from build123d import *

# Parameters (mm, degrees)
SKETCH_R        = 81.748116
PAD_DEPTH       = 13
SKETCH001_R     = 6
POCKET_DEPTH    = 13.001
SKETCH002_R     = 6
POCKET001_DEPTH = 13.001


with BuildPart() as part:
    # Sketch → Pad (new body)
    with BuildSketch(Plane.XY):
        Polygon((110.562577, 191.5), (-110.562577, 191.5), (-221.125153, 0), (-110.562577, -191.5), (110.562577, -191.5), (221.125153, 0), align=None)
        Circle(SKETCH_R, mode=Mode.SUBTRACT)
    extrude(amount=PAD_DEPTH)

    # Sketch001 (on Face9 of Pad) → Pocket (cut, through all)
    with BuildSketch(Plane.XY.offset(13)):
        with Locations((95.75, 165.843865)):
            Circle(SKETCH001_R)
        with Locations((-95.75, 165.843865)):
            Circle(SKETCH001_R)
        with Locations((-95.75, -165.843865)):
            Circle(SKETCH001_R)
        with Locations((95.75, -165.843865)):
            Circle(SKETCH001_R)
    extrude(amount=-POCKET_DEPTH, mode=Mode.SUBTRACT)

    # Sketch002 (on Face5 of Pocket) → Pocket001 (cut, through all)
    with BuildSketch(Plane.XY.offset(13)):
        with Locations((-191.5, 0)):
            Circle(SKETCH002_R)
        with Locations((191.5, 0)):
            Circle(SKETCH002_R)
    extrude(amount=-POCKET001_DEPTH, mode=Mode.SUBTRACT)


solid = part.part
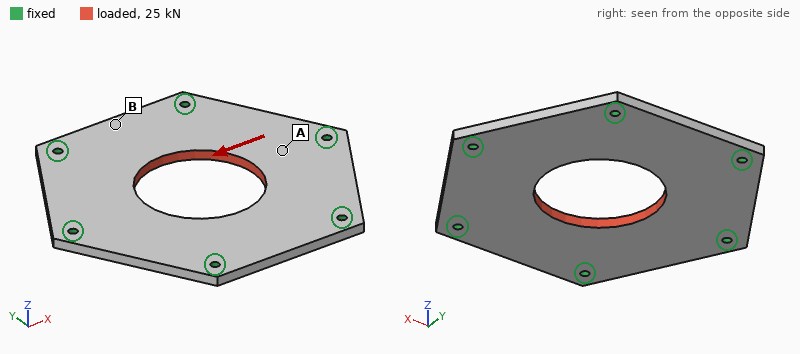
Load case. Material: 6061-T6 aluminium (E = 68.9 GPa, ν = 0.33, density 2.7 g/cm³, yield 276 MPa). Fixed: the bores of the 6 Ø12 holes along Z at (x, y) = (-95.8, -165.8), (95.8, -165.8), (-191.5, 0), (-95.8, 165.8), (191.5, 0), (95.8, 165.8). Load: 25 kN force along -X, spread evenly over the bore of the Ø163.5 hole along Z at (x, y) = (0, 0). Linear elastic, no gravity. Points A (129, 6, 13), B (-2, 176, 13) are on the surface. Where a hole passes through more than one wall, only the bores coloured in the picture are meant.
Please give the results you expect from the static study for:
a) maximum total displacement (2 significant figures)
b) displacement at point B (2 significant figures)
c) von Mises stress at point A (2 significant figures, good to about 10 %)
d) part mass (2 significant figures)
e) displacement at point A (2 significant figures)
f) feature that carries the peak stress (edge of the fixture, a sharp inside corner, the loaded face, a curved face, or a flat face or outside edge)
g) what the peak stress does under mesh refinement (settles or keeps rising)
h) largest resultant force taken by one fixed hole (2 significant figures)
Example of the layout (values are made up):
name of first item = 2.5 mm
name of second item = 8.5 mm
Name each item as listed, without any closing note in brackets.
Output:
maximum total displacement = 11 µm
displacement at point B = 2.5 µm
von Mises stress at point A = 5.9 MPa
part mass = 3.7 kg
displacement at point A = 7.4 µm
feature that carries the peak stress = edge of the fixture
what the peak stress does under mesh refinement = keeps rising
largest resultant force taken by one fixed hole = 6.0 kN
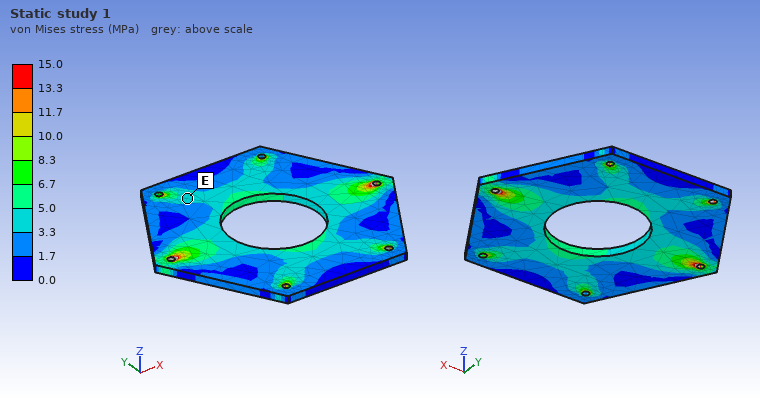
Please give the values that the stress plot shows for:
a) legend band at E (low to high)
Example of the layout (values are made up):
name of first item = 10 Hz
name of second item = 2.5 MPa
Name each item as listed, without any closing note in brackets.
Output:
legend band at E = 3.3 to 5.0 MPa
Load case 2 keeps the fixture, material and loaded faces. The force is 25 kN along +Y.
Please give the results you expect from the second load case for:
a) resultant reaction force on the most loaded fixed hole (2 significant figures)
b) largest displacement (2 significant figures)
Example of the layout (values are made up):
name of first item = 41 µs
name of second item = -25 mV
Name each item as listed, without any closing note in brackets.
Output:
resultant reaction force on the most loaded fixed hole = 5.4 kN
largest displacement = 11 µm
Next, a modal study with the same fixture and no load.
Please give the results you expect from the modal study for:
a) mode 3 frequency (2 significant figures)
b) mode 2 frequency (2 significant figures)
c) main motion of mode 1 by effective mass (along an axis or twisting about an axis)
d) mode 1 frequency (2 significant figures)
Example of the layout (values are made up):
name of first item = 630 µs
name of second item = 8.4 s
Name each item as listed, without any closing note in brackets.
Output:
mode 3 frequency = 1300 Hz
mode 2 frequency = 1300 Hz
main motion of mode 1 by effective mass = along Z
mode 1 frequency = 860 Hz
